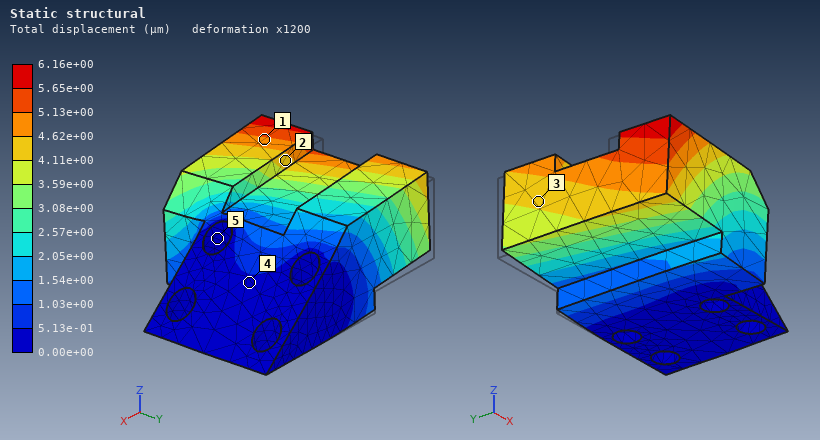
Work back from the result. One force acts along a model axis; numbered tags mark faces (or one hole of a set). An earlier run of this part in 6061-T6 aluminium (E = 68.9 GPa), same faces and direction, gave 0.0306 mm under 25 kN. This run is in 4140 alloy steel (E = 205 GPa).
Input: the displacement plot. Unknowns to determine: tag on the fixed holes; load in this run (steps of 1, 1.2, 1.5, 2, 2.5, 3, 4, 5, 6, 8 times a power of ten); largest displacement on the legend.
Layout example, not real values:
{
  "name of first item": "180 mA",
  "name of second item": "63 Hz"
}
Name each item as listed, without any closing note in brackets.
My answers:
{
  "tag on the fixed holes": "5",
  "load in this run": "15 kN",
  "largest displacement on the legend": "6.16e+00 µm"
}
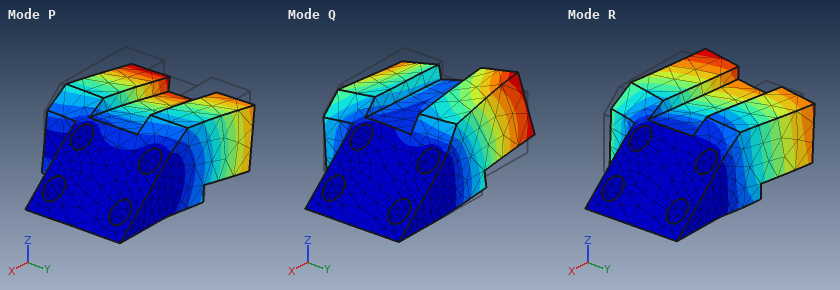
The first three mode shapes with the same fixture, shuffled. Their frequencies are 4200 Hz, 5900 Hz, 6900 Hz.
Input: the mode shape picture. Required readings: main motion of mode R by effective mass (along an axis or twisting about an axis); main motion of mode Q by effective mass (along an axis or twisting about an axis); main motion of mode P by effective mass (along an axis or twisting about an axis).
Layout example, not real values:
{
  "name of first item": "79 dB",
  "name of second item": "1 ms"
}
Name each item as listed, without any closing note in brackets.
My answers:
{
  "main motion of mode R by effective mass": "along Y",
  "main motion of mode Q by effective mass": "twisting about X",
  "main motion of mode P by effective mass": "along Z"
}
